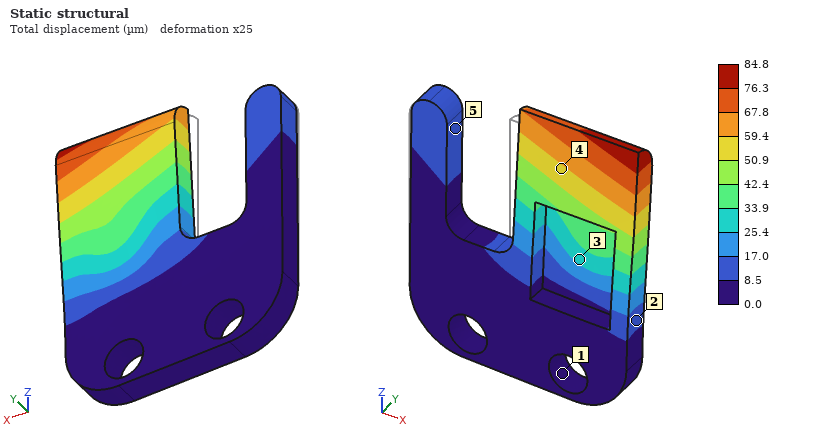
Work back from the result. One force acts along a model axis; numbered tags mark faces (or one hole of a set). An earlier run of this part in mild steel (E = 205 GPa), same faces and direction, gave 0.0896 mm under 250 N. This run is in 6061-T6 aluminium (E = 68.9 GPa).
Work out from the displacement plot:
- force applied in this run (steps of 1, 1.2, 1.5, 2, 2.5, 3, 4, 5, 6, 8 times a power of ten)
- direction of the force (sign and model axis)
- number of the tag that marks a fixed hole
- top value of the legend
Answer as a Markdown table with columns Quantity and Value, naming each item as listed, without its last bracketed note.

| Quantity | Value |
|---|---|
| force applied in this run | 80 N |
| direction of the force | +Y |
| number of the tag that marks a fixed hole | 1 |
| top value of the legend | 84.8 µm |
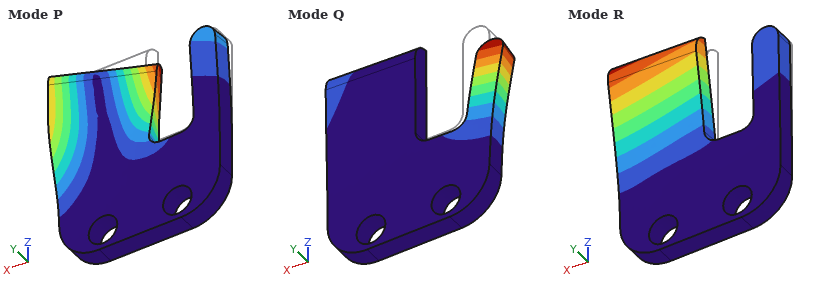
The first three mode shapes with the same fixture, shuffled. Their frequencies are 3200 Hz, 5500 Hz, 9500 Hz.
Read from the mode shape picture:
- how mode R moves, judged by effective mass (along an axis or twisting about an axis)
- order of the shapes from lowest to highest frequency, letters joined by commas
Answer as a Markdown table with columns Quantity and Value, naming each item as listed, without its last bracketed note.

| Quantity | Value |
|---|---|
| how mode R moves, judged by effective mass | along Y |
| order of the shapes from lowest to highest frequency, letters joined by commas | R, Q, P |
